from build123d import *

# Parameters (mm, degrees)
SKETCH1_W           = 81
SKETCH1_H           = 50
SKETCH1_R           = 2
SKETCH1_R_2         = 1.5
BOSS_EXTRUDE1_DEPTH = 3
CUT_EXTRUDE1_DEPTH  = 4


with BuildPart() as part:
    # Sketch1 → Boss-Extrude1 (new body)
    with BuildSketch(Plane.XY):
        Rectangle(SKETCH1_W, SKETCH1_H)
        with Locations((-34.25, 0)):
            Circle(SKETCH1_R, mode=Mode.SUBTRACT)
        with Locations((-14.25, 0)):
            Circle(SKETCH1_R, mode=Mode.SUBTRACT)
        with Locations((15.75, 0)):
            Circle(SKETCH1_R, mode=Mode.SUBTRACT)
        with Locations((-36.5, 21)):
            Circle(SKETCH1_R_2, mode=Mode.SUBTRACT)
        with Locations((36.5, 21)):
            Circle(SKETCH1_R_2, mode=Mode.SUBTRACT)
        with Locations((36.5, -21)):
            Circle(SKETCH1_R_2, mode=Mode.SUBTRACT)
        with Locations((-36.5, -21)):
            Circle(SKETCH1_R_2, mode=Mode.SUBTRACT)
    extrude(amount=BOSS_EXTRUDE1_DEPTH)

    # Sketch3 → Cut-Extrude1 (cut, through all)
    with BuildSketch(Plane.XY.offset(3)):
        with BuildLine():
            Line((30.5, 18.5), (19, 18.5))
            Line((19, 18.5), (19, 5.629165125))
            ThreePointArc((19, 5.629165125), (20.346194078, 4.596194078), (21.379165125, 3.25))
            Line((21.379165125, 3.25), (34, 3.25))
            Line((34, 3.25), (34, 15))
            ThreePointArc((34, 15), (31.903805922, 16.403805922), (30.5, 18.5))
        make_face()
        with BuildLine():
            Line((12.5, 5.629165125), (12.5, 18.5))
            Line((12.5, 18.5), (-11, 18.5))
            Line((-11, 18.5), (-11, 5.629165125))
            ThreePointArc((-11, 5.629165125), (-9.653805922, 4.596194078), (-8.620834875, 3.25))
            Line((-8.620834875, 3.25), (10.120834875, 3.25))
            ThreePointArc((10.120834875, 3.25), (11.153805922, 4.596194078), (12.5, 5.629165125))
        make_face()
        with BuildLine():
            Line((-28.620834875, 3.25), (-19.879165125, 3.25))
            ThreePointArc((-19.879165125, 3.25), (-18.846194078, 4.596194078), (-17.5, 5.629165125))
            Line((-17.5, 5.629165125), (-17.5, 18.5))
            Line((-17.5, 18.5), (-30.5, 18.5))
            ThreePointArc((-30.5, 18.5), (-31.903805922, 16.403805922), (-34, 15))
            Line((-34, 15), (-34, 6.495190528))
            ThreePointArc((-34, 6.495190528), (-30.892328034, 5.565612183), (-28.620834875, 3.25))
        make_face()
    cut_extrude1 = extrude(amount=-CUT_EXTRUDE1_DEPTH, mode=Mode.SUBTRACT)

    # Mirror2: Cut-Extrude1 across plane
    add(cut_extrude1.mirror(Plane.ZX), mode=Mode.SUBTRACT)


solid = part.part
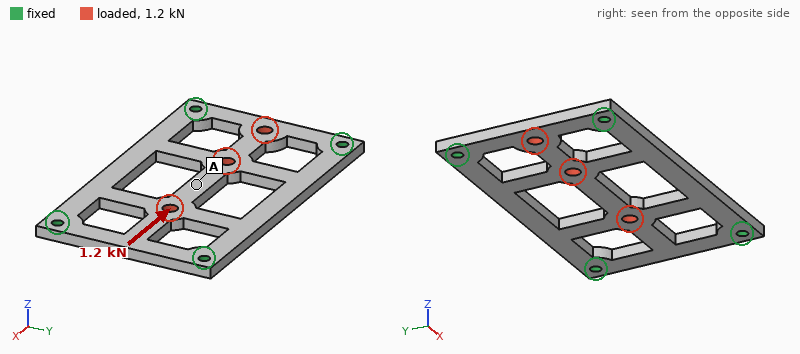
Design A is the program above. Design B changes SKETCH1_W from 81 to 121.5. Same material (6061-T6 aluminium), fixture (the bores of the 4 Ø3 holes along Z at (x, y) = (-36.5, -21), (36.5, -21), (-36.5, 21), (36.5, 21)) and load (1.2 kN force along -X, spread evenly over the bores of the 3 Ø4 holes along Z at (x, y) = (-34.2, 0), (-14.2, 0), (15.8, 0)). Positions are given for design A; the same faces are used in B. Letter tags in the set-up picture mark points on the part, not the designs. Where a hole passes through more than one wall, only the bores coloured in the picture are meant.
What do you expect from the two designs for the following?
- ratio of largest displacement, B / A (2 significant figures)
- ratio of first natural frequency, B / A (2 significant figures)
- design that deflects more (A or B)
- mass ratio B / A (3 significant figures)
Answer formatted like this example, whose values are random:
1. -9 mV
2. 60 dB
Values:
1. 0.40
2. 1.0
3. A
4. 1.85
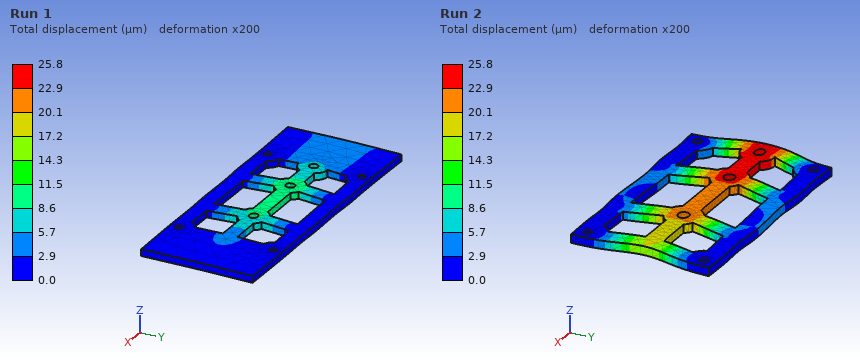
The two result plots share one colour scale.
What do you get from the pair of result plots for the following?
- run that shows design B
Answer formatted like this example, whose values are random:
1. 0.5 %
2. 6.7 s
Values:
1. Run 1
